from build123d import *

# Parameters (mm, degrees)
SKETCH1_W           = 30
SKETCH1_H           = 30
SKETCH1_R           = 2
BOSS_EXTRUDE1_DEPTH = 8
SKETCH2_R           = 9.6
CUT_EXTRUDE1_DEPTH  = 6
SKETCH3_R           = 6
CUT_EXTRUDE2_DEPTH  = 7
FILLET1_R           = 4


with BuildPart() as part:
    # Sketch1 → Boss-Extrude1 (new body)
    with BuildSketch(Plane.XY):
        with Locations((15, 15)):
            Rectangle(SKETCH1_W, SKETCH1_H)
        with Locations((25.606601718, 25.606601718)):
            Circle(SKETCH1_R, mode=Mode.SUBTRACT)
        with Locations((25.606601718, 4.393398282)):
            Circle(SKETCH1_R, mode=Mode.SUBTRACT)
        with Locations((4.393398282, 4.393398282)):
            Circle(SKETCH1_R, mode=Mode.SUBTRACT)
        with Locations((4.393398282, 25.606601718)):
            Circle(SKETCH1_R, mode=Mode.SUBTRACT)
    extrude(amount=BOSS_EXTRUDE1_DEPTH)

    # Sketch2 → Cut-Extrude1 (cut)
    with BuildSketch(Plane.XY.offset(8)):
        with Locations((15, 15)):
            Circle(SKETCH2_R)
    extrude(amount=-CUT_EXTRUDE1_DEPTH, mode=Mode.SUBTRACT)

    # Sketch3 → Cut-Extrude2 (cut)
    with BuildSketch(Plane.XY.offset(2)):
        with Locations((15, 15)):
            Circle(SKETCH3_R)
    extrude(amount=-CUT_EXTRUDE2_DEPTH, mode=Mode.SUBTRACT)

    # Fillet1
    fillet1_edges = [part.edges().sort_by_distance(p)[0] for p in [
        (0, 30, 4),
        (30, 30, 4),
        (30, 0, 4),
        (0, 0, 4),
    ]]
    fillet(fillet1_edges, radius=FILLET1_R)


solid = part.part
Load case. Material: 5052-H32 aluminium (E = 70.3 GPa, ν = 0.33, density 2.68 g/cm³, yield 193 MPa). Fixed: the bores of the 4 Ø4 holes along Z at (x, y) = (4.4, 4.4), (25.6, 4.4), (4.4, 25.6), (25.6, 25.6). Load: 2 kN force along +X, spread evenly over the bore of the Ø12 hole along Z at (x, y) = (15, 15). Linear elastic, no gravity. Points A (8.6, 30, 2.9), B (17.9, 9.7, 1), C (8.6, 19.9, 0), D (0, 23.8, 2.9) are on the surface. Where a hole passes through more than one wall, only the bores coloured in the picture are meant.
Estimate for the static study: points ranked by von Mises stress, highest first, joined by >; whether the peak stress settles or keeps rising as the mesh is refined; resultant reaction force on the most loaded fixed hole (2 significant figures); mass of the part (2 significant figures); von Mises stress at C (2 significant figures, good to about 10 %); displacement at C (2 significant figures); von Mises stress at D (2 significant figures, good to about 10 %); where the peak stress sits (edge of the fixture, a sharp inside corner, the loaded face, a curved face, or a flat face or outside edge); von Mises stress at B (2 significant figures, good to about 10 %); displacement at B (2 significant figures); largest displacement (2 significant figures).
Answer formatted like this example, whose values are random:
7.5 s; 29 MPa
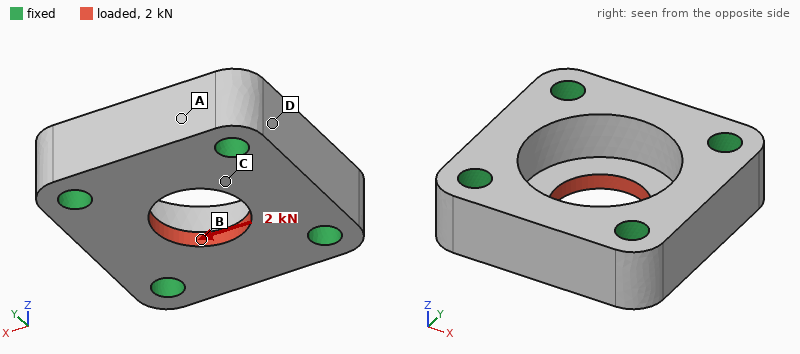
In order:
B > C > D > A; keeps rising; 520 N; 13 g; 24 MPa; 2.9 µm; 10 MPa; edge of the fixture; 45 MPa; 3.5 µm; 5.3 µm
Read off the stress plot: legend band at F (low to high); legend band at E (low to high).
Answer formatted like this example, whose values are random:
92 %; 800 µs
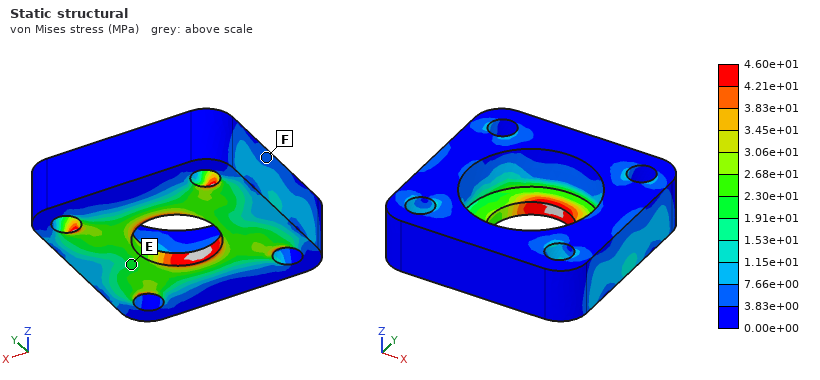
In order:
3.83e+00 to 7.66e+00 MPa; 1.91e+01 to 2.30e+01 MPa
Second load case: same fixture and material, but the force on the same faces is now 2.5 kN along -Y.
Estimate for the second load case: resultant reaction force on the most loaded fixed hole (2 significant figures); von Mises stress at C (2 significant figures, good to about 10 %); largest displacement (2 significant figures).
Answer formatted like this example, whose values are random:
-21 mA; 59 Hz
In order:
650 N; 30 MPa; 6.6 µm
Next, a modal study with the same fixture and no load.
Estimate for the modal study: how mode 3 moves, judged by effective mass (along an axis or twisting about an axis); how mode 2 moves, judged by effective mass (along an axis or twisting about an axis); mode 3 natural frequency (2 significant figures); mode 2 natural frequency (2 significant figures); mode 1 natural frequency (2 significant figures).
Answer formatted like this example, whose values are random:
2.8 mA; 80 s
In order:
twisting about Y; along Z; 66 kHz; 63 kHz; 57 kHz
